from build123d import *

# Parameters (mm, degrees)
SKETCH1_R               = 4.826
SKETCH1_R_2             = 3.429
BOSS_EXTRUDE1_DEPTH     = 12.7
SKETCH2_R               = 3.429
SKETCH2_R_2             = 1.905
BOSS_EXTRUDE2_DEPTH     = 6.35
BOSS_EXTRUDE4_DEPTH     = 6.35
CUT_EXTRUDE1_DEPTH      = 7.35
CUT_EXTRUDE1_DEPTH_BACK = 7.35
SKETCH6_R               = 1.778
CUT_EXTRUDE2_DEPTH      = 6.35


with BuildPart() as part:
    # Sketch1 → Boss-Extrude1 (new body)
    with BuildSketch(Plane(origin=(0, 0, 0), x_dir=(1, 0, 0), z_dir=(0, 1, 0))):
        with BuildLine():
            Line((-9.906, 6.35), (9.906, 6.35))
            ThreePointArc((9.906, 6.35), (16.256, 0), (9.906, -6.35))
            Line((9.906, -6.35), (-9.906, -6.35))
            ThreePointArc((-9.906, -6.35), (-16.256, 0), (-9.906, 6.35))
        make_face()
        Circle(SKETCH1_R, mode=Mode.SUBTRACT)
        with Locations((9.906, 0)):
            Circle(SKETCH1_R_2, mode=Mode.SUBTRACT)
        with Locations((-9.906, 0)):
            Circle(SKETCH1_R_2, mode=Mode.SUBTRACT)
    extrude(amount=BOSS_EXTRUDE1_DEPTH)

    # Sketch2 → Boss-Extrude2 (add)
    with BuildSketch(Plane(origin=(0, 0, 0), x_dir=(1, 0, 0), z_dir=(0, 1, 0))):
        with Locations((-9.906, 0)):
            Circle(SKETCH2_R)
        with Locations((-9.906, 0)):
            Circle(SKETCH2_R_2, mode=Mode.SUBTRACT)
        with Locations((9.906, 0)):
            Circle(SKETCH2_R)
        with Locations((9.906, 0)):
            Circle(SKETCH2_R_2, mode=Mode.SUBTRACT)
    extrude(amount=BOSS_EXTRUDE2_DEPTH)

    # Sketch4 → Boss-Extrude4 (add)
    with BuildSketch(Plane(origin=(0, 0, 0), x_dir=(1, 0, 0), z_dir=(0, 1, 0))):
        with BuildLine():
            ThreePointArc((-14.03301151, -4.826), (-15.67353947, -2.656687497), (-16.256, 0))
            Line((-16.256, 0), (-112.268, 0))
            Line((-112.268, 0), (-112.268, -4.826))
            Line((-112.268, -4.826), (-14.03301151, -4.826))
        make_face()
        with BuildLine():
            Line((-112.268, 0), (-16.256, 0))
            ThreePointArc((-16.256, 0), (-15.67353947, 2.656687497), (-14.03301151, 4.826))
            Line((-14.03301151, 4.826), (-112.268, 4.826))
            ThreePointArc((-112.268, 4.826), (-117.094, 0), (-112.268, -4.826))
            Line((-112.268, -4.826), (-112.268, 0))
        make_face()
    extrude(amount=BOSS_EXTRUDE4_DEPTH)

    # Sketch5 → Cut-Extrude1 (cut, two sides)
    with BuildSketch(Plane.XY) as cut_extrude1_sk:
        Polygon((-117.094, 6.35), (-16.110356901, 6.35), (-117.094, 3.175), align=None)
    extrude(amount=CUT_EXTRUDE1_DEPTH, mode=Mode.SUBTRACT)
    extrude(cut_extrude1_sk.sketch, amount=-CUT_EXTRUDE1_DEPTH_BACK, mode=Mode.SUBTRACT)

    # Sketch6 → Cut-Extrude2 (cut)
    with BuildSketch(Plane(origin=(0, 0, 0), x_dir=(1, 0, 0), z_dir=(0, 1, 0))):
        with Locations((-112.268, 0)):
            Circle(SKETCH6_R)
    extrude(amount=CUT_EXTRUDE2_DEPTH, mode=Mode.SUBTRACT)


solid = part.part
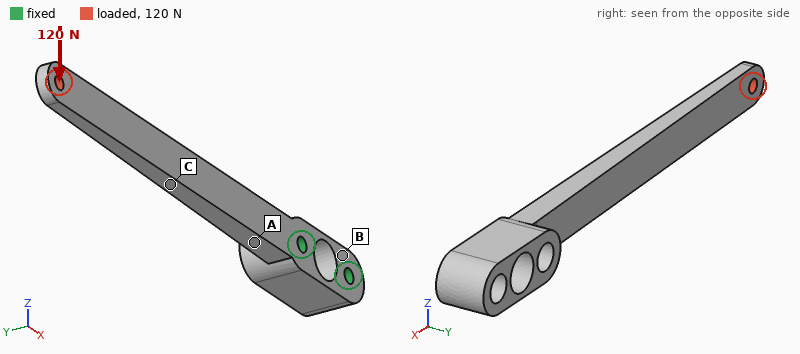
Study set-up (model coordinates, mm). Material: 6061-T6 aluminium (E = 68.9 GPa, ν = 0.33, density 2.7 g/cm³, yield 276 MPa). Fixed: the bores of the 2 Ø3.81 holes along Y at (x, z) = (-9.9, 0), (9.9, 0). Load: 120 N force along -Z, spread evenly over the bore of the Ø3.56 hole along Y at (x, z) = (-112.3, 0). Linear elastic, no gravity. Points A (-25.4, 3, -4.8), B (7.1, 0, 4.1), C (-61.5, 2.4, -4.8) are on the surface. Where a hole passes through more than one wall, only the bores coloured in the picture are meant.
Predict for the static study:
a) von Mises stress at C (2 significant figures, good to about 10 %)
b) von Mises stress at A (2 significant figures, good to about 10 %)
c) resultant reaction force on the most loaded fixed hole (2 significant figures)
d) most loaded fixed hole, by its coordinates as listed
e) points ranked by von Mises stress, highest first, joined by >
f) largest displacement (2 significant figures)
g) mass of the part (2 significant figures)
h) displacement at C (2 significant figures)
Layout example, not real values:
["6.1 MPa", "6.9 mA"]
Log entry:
["80 MPa", "110 MPa", "280 N", "(-9.9, 0)", "A > C > B", "1.6 mm", "21 g", "0.45 mm"]
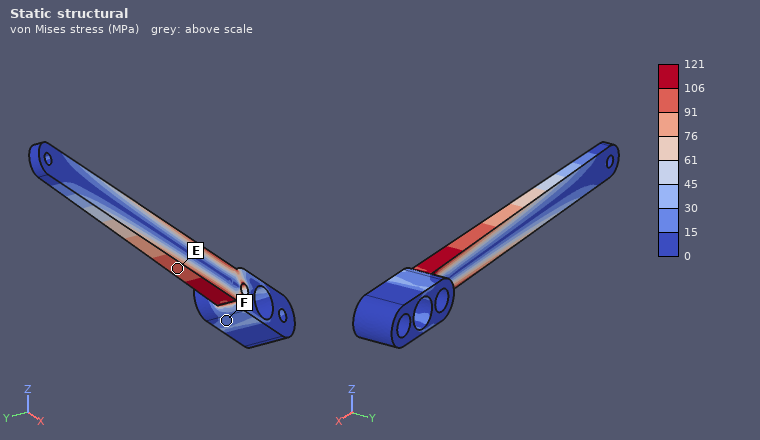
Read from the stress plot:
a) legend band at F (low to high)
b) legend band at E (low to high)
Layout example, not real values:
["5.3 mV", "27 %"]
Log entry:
["15 to 30 MPa", "91 to 106 MPa"]
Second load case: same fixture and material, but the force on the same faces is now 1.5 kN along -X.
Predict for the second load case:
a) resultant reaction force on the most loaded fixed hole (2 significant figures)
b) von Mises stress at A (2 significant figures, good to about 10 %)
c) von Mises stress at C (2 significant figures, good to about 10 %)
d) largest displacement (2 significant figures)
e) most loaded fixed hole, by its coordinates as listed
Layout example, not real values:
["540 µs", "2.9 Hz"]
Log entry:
["1.5 kN", "26 MPa", "32 MPa", "0.93 mm", "(-9.9, 0)"]
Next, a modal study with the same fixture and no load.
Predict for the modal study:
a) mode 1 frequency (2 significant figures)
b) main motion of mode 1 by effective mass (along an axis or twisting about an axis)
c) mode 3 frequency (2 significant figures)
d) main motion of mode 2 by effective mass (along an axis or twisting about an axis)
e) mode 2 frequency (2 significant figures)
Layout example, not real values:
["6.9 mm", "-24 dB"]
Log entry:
["540 Hz", "along Y", "2600 Hz", "along Z", "870 Hz"]
